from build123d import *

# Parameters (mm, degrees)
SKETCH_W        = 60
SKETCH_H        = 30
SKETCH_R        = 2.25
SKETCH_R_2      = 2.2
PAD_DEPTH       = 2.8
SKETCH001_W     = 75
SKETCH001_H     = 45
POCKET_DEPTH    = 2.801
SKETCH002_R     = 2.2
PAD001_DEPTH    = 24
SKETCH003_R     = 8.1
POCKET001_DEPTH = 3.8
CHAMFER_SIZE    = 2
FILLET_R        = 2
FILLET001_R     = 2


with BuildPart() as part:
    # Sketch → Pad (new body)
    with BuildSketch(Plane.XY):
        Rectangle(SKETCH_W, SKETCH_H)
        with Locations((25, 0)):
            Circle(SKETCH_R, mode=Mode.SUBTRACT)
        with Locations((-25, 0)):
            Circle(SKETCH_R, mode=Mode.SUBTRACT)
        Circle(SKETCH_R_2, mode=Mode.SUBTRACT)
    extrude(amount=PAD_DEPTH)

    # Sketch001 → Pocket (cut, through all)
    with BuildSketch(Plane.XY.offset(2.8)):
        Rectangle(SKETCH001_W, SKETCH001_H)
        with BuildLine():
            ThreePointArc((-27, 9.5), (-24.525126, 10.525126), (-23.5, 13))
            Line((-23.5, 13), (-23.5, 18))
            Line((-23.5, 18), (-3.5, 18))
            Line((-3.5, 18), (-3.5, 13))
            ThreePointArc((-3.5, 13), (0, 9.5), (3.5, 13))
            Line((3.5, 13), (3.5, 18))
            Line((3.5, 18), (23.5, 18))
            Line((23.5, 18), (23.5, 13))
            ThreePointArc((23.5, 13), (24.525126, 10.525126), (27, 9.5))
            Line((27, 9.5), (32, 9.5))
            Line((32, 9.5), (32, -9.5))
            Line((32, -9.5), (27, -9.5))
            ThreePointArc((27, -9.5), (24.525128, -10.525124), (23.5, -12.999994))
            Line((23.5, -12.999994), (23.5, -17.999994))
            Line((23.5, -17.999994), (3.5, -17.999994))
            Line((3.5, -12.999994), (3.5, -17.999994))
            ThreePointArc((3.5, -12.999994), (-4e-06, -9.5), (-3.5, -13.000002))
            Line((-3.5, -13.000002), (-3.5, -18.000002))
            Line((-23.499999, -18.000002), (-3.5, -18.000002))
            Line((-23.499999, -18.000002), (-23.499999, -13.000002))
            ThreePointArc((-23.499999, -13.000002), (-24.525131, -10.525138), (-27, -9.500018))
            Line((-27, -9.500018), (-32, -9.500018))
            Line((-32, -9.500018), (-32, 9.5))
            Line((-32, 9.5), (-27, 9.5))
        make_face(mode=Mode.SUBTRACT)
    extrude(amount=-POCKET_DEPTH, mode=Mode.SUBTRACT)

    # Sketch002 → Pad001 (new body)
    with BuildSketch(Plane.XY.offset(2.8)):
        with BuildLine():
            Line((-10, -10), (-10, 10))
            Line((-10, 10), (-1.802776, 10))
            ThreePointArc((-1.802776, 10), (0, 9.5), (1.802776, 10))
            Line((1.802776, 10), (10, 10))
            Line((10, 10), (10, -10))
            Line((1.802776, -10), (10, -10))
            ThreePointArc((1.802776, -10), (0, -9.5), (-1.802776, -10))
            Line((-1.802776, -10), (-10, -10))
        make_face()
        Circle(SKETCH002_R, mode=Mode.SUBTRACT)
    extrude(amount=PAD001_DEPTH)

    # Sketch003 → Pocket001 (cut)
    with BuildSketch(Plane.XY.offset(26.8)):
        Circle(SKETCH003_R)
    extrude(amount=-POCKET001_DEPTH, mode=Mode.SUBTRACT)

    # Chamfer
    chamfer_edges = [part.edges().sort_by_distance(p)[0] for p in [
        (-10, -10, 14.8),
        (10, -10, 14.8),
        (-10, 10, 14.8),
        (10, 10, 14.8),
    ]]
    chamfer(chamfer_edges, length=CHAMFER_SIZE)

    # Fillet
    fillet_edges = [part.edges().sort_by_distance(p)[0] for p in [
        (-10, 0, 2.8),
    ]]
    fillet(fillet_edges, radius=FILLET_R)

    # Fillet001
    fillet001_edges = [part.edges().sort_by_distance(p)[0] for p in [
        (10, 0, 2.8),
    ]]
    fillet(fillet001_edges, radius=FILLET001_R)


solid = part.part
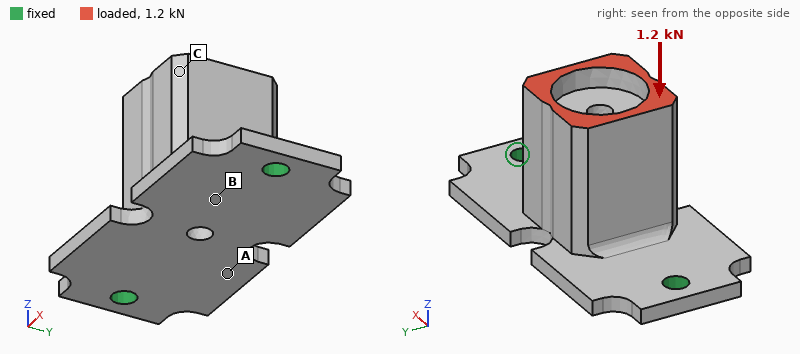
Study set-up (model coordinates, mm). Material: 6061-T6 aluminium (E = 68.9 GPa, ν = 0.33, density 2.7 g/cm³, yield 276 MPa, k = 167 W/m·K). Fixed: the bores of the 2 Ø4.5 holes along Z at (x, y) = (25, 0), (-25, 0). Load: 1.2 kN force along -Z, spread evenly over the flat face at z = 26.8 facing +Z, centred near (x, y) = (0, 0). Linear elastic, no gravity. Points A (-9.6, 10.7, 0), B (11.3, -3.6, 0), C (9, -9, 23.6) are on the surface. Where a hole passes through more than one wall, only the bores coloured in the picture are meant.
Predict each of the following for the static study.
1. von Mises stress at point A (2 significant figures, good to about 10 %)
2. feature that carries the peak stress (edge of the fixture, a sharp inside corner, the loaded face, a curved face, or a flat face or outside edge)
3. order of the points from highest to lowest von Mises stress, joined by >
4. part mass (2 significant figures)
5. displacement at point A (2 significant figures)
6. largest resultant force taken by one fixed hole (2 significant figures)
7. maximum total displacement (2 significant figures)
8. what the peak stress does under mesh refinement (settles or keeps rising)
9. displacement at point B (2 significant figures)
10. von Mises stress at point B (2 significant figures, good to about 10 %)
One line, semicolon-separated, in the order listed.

50 MPa; edge of the fixture; B > A > C; 34 g; 70 µm; 680 N; 78 µm; keeps rising; 66 µm; 86 MPa
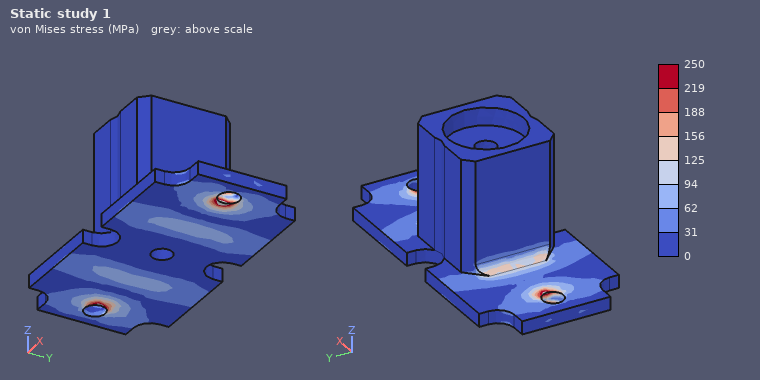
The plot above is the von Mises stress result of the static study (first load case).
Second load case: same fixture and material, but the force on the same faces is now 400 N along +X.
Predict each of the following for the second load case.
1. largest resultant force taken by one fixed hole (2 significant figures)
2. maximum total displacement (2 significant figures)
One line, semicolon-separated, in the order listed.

340 N; 55 µm
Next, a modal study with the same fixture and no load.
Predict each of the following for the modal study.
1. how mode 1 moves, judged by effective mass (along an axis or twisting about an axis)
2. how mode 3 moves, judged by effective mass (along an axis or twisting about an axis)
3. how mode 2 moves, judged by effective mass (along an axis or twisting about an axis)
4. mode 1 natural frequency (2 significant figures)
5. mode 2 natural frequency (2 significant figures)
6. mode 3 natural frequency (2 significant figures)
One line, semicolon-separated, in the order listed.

along Y; along X; along Z; 1800 Hz; 3800 Hz; 4900 Hz
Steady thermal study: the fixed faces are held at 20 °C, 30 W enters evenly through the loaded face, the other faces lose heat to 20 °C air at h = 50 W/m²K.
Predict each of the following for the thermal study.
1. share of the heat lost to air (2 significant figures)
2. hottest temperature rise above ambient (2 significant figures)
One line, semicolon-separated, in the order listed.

17 %; 34 K
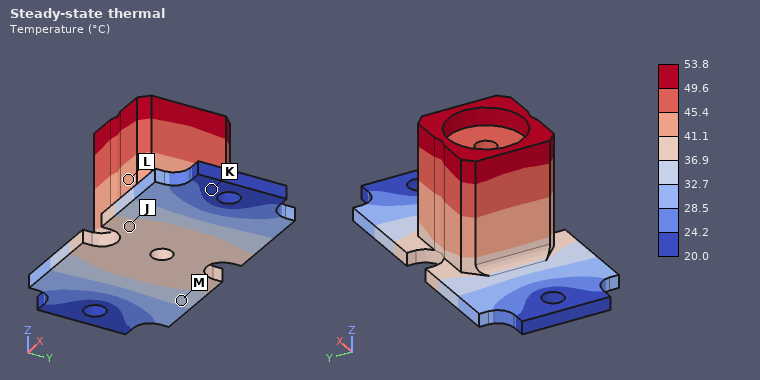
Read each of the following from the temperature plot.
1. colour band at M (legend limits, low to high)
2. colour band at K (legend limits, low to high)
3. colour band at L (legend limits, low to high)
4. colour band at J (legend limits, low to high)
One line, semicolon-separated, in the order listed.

32.7 to 36.9 °C; 20.0 to 24.2 °C; 41.1 to 45.4 °C; 36.9 to 41.1 °C
